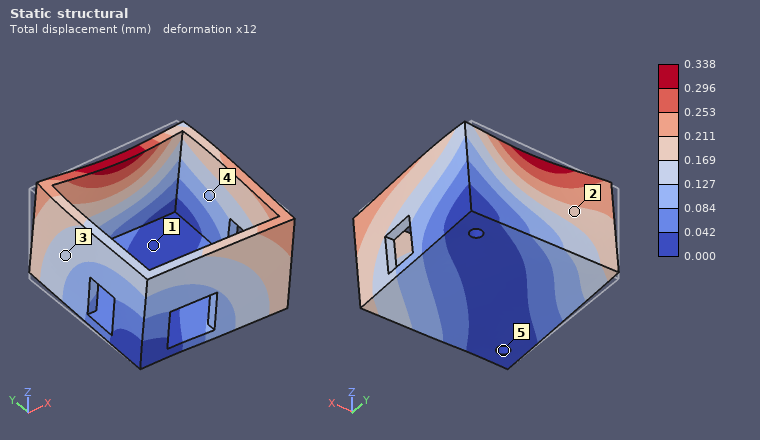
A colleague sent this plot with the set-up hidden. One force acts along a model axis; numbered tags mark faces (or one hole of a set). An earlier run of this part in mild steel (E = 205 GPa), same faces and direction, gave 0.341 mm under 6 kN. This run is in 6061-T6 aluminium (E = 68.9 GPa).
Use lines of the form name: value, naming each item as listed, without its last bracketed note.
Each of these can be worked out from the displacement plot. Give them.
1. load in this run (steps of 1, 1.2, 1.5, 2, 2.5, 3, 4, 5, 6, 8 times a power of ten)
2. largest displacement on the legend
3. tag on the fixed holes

load in this run: 2 kN
largest displacement on the legend: 0.338 mm
tag on the fixed holes: 5
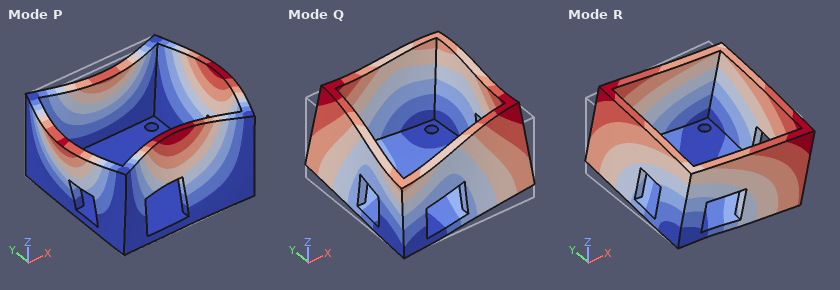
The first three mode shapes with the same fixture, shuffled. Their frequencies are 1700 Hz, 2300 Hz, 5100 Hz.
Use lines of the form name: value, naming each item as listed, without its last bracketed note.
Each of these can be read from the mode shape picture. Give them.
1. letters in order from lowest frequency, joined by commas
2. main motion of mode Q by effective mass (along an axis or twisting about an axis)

letters in order from lowest frequency, joined by commas: R, Q, P
main motion of mode Q by effective mass: along Z
